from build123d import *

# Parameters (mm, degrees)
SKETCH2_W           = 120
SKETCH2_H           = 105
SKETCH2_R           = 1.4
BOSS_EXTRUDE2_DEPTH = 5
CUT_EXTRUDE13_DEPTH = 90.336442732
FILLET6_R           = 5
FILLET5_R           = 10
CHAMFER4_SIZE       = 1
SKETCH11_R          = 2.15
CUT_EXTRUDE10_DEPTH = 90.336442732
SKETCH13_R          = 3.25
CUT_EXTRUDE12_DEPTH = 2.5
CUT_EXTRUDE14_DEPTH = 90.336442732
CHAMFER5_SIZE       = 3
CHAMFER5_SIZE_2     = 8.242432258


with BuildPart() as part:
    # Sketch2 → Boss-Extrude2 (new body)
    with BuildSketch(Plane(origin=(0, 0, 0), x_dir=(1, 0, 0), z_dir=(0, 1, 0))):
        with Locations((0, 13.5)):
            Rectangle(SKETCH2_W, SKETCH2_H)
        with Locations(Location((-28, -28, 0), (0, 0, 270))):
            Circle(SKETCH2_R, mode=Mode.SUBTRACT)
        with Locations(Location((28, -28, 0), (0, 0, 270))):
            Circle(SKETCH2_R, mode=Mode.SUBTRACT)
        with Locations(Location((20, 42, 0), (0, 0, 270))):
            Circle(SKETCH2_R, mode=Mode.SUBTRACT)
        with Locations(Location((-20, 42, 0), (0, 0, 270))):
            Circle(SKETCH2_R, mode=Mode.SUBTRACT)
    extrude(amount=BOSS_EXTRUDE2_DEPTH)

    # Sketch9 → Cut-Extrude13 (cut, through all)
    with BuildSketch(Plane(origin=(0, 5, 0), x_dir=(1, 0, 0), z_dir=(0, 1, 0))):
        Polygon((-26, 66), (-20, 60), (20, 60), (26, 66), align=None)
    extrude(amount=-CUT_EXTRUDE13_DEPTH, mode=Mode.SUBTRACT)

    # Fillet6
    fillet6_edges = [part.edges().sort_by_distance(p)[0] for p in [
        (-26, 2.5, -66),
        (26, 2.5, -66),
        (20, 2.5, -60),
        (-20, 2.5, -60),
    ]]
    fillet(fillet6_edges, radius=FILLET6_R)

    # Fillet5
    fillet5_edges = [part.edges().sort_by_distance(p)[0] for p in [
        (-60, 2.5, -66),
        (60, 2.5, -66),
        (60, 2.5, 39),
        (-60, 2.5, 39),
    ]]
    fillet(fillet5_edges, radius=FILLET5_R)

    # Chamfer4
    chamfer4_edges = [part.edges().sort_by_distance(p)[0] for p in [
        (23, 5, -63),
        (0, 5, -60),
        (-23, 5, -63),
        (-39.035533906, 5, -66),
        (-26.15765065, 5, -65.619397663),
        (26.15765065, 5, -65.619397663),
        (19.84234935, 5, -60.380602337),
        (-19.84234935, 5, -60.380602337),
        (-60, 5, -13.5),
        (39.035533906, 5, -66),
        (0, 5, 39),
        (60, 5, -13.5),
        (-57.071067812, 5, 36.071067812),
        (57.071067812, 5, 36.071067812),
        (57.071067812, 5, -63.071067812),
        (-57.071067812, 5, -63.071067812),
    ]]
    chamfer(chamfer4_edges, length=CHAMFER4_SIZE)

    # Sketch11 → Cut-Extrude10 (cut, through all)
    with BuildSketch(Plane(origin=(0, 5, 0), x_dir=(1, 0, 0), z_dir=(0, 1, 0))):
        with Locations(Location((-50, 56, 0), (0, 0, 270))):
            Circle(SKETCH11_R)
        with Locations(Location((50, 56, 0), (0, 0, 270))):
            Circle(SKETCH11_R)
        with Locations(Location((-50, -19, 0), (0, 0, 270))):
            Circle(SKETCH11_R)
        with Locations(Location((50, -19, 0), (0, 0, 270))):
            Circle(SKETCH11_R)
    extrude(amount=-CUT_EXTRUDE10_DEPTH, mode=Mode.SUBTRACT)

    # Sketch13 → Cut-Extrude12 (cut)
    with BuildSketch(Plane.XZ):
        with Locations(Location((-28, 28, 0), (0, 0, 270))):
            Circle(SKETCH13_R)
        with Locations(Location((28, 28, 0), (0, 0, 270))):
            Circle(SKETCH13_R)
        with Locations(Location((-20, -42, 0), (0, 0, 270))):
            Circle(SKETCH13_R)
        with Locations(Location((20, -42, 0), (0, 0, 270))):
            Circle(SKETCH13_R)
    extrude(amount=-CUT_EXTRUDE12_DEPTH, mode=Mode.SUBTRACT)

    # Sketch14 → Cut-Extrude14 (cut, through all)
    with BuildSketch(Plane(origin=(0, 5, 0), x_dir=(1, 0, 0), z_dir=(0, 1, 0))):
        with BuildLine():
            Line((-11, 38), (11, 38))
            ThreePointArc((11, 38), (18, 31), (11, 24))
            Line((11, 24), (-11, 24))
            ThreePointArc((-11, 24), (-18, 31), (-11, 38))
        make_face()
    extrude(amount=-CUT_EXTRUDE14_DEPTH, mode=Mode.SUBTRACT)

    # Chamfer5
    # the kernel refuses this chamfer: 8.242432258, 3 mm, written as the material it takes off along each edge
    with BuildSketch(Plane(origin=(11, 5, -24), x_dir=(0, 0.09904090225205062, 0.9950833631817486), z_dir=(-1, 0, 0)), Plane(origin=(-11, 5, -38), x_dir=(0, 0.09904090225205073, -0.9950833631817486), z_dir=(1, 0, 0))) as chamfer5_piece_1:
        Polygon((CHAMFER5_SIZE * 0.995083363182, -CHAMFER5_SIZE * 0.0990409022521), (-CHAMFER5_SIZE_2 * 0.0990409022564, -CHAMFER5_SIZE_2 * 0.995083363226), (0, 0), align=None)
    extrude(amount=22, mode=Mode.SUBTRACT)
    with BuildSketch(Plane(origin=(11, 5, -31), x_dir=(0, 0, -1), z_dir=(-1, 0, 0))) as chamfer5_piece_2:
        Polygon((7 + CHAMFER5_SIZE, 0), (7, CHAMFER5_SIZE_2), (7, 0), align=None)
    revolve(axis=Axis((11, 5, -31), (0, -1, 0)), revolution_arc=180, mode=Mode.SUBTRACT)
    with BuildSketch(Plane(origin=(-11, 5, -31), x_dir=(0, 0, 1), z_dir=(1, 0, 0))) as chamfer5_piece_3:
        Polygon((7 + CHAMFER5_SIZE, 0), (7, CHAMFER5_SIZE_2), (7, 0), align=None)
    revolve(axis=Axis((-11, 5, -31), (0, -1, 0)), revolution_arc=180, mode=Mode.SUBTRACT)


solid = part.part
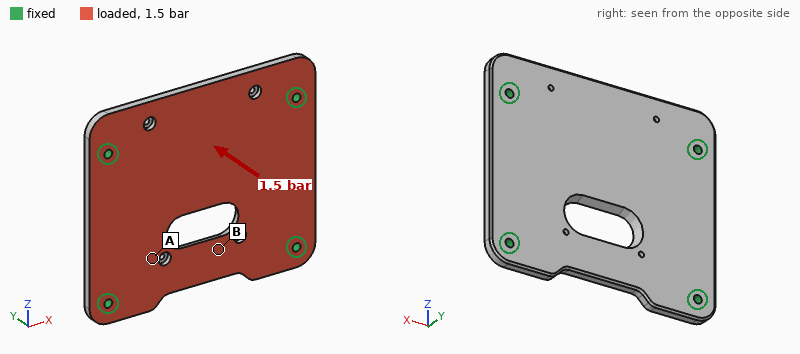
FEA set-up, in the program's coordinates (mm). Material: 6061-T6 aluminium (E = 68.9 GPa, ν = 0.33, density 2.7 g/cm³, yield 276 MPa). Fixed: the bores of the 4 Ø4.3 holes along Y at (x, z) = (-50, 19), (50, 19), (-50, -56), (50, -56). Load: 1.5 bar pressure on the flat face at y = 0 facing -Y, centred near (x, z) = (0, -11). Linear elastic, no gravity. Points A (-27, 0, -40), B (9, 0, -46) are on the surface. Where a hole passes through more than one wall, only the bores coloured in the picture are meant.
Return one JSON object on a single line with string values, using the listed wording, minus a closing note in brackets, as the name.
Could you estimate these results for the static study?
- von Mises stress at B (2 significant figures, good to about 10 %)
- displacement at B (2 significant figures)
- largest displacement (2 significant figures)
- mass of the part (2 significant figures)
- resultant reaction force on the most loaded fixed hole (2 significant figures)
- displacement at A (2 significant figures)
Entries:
{"von Mises stress at B": "16 MPa", "displacement at B": "0.081 mm", "largest displacement": "0.11 mm", "mass of the part": "150 g", "resultant reaction force on the most loaded fixed hole": "500 N", "displacement at A": "0.059 mm"}
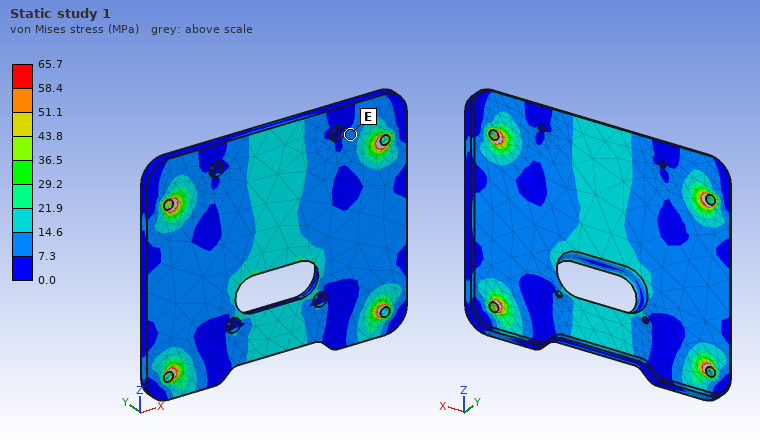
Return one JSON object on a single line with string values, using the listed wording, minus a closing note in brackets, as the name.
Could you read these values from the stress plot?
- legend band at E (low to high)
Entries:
{"legend band at E": "7.3 to 14.6 MPa"}
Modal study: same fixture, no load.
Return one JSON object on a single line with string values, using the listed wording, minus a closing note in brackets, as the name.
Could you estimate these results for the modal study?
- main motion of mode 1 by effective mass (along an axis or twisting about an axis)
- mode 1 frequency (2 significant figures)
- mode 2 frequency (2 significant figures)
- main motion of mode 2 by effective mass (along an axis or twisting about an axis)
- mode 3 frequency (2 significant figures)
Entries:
{"main motion of mode 1 by effective mass": "along Y", "mode 1 frequency": "2100 Hz", "mode 2 frequency": "2800 Hz", "main motion of mode 2 by effective mass": "twisting about X", "mode 3 frequency": "3800 Hz"}
